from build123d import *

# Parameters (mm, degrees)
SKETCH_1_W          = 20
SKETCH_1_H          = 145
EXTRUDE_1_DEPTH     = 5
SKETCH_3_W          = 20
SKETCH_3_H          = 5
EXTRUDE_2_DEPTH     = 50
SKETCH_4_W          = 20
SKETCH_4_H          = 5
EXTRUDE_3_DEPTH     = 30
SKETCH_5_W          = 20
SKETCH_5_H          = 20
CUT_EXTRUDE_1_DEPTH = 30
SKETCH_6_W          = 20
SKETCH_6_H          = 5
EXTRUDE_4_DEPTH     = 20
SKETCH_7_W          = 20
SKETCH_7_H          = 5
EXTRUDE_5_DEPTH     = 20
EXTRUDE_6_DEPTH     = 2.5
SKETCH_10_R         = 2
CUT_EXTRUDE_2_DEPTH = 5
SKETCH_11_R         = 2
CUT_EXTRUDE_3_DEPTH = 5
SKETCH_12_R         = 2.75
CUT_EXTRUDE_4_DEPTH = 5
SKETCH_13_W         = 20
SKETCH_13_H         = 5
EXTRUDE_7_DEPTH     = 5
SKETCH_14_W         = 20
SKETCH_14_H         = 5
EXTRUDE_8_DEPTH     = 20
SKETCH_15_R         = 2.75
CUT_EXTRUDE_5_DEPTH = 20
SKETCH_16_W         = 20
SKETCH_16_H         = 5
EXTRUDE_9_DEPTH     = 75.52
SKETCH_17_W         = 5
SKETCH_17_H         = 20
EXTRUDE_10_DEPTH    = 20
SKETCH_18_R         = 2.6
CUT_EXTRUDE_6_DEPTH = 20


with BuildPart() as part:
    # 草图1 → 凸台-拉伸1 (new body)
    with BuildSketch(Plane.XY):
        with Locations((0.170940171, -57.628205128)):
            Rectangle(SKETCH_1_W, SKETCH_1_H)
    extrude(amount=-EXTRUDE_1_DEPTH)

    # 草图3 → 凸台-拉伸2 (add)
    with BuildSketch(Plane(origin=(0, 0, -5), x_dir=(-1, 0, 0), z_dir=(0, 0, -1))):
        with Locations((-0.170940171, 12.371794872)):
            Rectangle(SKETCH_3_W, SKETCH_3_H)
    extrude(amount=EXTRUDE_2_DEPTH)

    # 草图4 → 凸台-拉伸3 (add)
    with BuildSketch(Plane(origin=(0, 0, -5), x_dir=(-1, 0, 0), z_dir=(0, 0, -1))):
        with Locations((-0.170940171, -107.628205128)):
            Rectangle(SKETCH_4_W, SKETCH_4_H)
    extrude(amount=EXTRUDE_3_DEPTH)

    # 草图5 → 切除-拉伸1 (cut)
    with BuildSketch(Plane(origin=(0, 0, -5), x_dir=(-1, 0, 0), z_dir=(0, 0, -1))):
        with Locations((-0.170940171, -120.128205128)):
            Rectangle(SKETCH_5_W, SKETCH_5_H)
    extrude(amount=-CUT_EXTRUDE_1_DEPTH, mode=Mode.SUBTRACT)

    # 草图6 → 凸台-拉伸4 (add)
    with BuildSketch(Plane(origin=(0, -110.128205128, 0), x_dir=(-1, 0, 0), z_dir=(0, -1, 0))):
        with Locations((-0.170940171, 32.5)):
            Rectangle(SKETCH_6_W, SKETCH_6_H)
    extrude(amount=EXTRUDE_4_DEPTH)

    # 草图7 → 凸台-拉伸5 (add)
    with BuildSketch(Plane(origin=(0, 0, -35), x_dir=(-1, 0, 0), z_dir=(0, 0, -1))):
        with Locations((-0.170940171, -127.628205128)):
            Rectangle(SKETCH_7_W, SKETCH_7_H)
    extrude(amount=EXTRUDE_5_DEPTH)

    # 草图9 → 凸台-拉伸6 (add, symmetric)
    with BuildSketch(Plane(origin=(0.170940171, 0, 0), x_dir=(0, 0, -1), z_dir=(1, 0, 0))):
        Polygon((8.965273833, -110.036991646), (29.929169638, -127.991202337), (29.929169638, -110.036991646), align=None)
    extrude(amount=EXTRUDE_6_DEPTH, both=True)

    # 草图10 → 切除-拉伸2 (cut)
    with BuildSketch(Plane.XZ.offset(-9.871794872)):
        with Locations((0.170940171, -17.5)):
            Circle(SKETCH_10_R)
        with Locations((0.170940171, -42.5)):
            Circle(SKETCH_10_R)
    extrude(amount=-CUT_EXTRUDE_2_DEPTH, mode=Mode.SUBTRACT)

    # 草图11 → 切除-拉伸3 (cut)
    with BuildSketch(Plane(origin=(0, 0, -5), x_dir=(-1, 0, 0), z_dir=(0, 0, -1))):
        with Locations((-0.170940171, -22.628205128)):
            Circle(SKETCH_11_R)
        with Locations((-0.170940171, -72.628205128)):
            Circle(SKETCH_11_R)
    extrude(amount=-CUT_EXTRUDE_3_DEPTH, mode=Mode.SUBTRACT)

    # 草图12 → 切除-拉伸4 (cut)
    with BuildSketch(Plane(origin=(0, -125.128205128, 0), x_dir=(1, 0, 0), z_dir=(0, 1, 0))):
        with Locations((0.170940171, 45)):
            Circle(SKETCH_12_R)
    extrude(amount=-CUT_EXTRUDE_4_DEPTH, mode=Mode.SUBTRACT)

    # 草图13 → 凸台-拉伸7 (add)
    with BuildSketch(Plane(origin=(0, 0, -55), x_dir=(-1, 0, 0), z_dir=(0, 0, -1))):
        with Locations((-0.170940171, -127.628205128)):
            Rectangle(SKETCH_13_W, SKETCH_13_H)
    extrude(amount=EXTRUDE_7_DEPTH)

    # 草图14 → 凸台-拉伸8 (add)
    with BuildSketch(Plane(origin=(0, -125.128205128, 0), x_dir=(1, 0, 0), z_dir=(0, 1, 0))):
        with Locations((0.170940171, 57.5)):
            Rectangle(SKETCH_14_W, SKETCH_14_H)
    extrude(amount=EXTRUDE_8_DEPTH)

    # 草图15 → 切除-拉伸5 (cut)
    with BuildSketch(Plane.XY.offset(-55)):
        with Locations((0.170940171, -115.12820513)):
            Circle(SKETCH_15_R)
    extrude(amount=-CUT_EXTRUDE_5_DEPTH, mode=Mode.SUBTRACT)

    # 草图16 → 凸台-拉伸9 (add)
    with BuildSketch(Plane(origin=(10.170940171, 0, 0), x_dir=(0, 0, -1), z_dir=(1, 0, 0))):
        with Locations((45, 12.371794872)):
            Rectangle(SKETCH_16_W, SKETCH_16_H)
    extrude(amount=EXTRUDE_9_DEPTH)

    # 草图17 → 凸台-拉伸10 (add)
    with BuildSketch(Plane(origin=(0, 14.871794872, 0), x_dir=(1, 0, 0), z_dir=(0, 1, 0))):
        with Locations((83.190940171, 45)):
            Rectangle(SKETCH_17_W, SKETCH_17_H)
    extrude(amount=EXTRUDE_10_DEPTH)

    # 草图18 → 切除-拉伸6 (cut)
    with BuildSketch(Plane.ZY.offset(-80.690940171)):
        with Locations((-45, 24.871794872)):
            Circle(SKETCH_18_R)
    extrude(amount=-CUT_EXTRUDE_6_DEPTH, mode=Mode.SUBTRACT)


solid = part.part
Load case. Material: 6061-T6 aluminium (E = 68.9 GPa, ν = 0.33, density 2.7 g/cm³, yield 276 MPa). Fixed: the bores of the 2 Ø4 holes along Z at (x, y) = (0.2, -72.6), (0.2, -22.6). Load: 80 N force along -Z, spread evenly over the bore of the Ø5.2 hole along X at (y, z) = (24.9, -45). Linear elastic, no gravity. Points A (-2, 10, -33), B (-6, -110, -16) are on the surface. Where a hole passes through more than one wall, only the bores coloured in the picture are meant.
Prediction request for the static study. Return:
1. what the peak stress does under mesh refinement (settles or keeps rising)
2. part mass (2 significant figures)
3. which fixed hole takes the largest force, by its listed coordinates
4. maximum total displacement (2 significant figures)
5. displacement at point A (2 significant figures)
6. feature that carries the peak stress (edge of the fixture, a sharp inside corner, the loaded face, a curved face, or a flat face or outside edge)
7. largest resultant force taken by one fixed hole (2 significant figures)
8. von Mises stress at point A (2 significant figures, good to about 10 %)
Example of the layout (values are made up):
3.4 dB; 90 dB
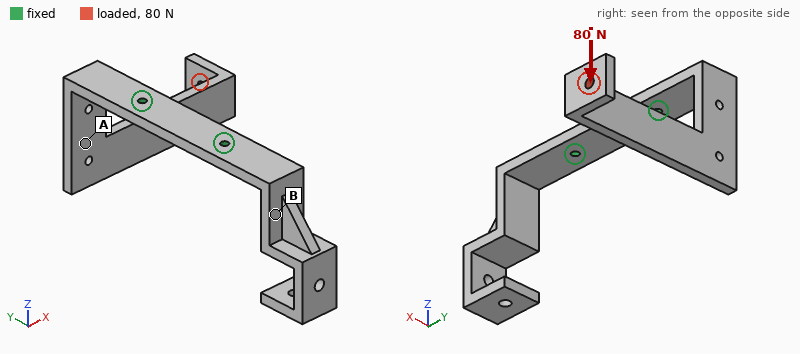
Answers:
keeps rising; 100 g; (0.2, -22.6); 1.7 mm; 0.42 mm; edge of the fixture; 89 N; 16 MPa
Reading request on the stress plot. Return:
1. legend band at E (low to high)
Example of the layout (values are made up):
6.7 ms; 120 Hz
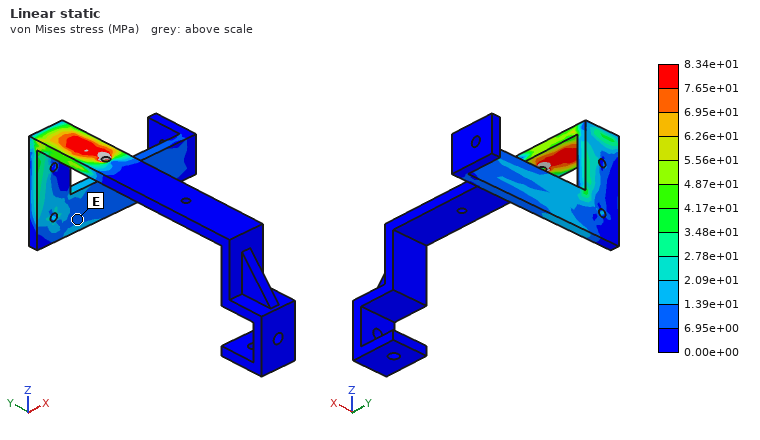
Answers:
6.95e+00 to 1.39e+01 MPa
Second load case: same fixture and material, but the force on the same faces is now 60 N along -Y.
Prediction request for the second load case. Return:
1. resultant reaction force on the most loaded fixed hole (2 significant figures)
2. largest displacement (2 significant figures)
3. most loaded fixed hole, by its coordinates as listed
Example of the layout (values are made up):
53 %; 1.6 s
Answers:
91 N; 2.2 mm; (0.2, -22.6)
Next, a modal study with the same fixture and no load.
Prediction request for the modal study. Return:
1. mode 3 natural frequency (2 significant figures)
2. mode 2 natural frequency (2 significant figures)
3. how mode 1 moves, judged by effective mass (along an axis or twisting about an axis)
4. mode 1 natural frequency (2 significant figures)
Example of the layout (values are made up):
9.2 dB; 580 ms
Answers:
380 Hz; 300 Hz; along Y; 230 Hz
